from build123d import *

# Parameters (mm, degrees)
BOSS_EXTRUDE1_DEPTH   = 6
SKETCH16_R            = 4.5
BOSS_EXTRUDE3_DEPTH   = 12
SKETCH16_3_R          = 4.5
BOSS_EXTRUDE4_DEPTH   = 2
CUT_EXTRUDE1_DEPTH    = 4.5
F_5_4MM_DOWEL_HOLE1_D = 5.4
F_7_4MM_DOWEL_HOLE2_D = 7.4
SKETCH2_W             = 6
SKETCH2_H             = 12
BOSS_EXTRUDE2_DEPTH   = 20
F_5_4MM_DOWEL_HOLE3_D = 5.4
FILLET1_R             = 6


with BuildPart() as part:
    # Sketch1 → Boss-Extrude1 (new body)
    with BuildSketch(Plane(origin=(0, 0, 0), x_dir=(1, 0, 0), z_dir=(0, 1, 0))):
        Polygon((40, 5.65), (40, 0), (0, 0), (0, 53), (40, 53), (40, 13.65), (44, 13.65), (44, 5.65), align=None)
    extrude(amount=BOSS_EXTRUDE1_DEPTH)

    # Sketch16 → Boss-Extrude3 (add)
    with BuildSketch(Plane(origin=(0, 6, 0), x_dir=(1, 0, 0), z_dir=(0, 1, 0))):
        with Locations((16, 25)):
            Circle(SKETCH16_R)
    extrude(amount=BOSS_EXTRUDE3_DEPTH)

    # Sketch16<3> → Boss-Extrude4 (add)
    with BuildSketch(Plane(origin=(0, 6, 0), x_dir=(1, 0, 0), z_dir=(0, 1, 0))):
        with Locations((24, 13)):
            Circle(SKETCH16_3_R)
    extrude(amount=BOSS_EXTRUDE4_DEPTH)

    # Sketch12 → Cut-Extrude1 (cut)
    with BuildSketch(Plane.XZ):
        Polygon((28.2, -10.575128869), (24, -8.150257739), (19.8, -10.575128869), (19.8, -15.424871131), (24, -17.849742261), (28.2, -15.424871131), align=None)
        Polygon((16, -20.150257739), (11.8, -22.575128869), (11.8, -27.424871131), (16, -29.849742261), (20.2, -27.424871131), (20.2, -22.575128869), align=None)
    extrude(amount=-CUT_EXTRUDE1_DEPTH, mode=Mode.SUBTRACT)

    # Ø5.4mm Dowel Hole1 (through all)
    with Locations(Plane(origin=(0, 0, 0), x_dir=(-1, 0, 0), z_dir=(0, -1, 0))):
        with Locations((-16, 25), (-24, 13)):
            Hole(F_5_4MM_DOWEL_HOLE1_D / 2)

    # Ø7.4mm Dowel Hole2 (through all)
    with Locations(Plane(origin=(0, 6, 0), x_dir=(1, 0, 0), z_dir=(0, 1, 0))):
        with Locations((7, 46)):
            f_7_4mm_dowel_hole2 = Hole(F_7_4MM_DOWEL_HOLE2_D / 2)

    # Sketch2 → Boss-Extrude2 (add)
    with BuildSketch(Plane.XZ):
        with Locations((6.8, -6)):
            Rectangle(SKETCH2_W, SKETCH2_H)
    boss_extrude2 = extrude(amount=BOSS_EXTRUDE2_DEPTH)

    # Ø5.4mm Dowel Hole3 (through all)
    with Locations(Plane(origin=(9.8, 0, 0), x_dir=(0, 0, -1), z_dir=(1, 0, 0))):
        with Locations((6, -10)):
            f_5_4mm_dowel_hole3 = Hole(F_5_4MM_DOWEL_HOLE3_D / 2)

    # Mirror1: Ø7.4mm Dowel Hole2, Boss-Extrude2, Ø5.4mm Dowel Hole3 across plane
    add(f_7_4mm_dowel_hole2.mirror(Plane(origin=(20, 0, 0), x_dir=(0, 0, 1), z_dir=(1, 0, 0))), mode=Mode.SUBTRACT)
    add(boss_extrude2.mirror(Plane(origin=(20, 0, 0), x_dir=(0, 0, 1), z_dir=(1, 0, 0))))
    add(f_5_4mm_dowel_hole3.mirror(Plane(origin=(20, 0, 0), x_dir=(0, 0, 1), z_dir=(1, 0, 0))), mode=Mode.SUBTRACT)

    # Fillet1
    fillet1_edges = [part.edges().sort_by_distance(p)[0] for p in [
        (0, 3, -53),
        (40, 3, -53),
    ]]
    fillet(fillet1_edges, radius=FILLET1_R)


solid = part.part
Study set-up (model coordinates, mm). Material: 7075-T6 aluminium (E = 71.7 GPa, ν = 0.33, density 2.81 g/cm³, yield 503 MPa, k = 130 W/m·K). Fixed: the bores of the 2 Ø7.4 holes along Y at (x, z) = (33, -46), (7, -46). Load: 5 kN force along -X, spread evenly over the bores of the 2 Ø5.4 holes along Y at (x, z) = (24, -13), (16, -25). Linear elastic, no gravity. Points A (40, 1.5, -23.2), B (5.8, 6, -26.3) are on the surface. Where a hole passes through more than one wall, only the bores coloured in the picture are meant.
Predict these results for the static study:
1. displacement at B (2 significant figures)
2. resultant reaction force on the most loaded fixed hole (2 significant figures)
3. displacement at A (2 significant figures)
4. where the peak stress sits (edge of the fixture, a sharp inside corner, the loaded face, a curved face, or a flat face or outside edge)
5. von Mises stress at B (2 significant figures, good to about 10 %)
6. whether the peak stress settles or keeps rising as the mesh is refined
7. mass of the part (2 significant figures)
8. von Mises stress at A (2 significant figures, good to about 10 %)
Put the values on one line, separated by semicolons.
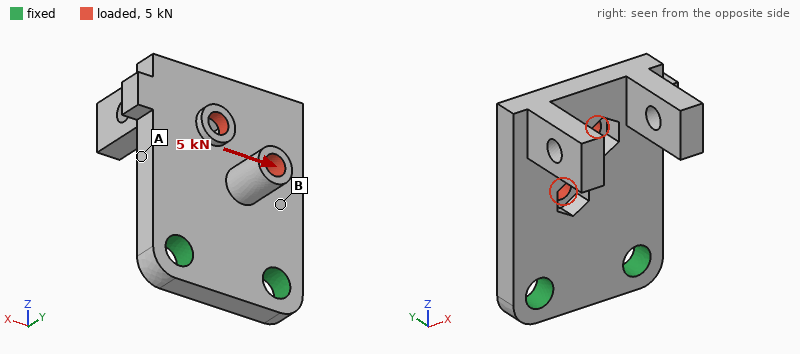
0.066 mm; 4.6 kN; 0.078 mm; a sharp inside corner; 100 MPa; keeps rising; 42 g; 37 MPa
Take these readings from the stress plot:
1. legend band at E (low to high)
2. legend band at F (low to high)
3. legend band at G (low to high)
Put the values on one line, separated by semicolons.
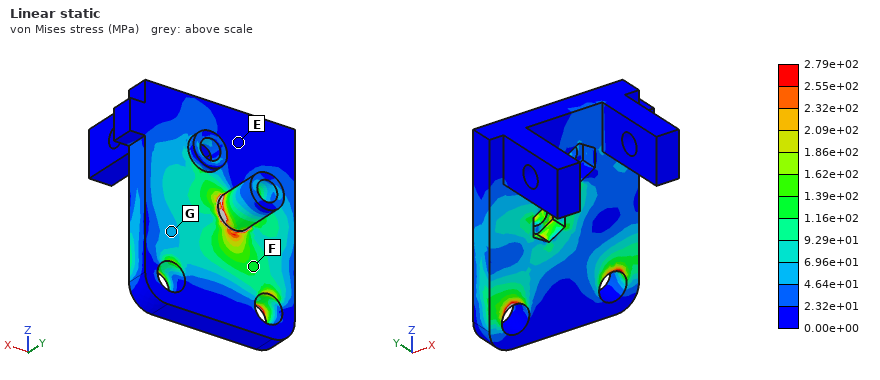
0.00e+00 to 2.32e+01 MPa; 1.16e+02 to 1.39e+02 MPa; 4.64e+01 to 6.96e+01 MPa
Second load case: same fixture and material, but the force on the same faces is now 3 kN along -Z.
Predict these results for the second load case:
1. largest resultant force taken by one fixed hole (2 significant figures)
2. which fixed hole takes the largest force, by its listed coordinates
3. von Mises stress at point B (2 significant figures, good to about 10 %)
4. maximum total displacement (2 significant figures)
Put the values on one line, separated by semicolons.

1.8 kN; (7, -46); 76 MPa; 0.36 mm
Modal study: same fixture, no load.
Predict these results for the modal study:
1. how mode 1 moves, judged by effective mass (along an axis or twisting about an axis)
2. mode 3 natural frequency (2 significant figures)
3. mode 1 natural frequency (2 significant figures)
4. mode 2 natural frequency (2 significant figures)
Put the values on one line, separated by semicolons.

along Y; 6300 Hz; 1800 Hz; 3500 Hz
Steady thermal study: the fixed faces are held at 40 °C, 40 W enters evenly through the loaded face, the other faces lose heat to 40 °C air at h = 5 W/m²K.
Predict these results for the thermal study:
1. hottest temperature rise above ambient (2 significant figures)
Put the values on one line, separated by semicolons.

71 K
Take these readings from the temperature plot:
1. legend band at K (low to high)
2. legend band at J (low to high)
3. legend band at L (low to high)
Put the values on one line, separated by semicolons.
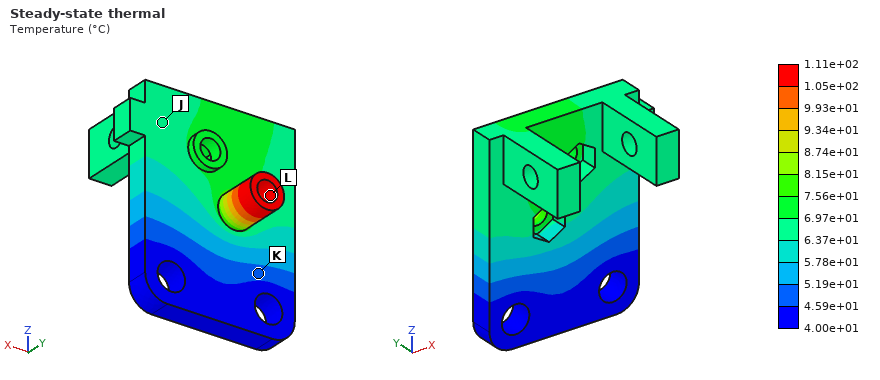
4.59e+01 to 5.19e+01 °C; 6.37e+01 to 6.97e+01 °C; 1.05e+02 to 1.11e+02 °C
